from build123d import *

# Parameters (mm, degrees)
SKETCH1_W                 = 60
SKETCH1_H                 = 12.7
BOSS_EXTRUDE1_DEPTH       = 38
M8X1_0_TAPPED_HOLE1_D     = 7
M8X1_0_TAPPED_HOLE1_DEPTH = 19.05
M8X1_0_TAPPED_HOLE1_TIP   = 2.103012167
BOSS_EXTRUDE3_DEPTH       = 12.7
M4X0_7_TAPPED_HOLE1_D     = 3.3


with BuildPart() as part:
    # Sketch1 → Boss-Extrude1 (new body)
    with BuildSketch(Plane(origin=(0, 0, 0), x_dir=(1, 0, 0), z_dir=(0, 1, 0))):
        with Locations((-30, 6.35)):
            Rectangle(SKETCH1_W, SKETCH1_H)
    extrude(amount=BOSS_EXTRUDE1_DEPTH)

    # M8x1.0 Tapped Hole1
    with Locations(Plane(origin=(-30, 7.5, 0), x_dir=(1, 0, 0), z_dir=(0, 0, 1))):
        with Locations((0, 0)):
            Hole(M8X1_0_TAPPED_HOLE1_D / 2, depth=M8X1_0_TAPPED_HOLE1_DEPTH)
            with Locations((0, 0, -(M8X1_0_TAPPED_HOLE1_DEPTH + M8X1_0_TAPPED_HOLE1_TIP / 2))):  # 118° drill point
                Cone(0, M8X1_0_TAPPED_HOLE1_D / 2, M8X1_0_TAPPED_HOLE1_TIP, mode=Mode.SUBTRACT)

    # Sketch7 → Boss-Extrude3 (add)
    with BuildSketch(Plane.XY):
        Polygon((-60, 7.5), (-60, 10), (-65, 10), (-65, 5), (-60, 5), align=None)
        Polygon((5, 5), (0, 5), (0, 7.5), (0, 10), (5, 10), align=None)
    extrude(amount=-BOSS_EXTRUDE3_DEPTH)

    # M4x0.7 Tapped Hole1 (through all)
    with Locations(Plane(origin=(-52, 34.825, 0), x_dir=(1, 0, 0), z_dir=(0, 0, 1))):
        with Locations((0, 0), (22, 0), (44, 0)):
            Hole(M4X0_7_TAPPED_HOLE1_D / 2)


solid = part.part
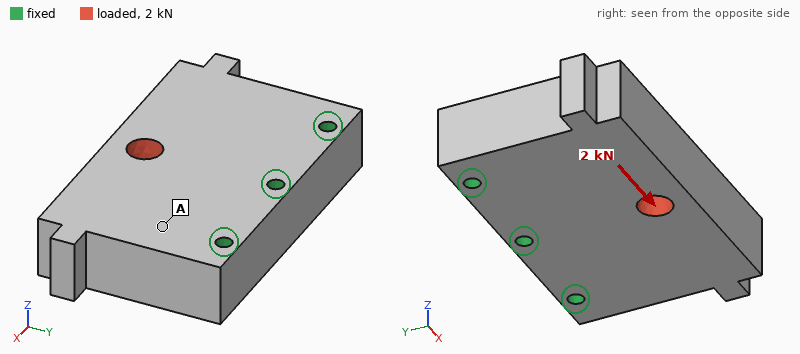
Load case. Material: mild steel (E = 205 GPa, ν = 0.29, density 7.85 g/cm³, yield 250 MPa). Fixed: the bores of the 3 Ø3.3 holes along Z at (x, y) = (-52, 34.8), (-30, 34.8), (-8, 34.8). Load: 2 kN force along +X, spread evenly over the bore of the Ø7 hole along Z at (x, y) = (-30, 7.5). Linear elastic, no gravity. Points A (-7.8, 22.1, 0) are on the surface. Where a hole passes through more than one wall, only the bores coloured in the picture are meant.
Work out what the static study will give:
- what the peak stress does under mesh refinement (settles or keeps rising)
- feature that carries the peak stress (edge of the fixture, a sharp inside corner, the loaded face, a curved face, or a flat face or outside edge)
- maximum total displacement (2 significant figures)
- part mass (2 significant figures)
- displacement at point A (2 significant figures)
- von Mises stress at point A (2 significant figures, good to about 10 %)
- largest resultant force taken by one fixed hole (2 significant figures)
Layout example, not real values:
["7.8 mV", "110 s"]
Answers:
["keeps rising", "edge of the fixture", "2.1 µm", "230 g", "0.83 µm", "4.8 MPa", "1.3 kN"]
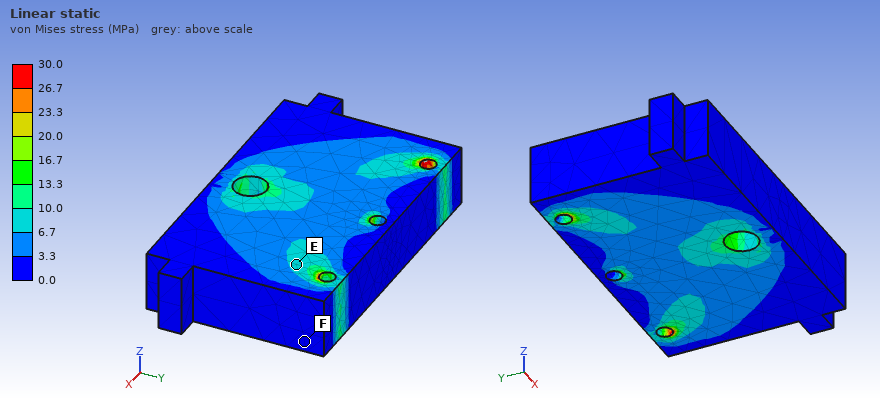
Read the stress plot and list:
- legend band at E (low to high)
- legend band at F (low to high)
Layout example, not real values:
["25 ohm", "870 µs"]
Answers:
["6.7 to 10.0 MPa", "0.0 to 3.3 MPa"]
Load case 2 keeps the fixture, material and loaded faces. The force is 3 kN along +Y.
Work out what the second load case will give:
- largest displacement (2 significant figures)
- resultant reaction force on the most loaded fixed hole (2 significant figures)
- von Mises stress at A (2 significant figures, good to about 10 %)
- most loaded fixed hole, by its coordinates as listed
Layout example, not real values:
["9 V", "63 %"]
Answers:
["1.9 µm", "1.4 kN", "3.1 MPa", "(-30, 34.8)"]
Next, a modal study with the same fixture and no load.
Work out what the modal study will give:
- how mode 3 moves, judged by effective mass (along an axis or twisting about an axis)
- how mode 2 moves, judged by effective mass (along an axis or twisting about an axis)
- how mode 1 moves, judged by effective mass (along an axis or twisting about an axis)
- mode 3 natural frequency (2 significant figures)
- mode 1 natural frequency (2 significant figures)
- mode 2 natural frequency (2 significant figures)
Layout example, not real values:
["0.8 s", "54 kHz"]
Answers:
["along X", "twisting about Y", "along Z", "16 kHz", "6600 Hz", "10 kHz"]
